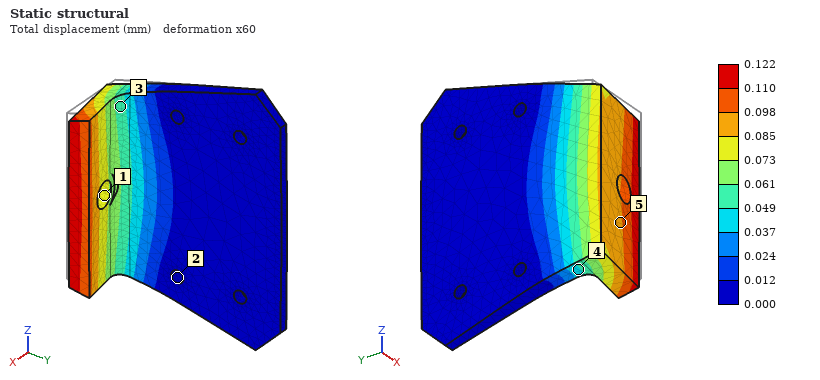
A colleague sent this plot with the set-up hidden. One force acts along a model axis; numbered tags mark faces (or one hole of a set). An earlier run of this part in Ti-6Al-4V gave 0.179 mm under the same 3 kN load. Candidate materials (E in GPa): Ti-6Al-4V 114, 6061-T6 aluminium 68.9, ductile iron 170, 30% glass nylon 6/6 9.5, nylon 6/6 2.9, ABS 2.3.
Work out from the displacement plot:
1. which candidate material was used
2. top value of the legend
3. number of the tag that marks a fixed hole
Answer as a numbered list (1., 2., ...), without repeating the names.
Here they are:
1. ductile iron
2. 0.122 mm
3. 2
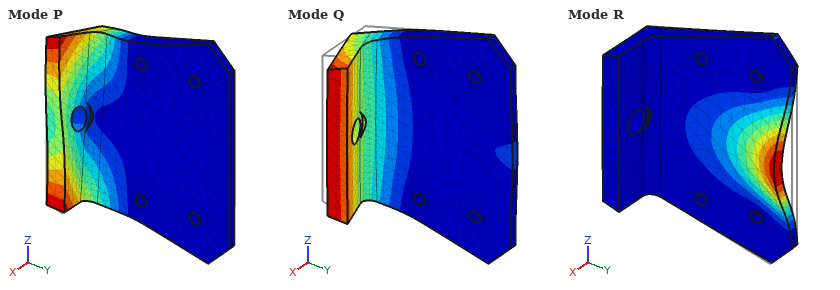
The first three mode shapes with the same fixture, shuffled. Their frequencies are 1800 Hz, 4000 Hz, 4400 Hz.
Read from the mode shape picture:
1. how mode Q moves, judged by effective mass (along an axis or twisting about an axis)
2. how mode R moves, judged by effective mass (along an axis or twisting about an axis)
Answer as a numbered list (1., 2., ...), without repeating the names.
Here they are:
1. along X
2. along X
